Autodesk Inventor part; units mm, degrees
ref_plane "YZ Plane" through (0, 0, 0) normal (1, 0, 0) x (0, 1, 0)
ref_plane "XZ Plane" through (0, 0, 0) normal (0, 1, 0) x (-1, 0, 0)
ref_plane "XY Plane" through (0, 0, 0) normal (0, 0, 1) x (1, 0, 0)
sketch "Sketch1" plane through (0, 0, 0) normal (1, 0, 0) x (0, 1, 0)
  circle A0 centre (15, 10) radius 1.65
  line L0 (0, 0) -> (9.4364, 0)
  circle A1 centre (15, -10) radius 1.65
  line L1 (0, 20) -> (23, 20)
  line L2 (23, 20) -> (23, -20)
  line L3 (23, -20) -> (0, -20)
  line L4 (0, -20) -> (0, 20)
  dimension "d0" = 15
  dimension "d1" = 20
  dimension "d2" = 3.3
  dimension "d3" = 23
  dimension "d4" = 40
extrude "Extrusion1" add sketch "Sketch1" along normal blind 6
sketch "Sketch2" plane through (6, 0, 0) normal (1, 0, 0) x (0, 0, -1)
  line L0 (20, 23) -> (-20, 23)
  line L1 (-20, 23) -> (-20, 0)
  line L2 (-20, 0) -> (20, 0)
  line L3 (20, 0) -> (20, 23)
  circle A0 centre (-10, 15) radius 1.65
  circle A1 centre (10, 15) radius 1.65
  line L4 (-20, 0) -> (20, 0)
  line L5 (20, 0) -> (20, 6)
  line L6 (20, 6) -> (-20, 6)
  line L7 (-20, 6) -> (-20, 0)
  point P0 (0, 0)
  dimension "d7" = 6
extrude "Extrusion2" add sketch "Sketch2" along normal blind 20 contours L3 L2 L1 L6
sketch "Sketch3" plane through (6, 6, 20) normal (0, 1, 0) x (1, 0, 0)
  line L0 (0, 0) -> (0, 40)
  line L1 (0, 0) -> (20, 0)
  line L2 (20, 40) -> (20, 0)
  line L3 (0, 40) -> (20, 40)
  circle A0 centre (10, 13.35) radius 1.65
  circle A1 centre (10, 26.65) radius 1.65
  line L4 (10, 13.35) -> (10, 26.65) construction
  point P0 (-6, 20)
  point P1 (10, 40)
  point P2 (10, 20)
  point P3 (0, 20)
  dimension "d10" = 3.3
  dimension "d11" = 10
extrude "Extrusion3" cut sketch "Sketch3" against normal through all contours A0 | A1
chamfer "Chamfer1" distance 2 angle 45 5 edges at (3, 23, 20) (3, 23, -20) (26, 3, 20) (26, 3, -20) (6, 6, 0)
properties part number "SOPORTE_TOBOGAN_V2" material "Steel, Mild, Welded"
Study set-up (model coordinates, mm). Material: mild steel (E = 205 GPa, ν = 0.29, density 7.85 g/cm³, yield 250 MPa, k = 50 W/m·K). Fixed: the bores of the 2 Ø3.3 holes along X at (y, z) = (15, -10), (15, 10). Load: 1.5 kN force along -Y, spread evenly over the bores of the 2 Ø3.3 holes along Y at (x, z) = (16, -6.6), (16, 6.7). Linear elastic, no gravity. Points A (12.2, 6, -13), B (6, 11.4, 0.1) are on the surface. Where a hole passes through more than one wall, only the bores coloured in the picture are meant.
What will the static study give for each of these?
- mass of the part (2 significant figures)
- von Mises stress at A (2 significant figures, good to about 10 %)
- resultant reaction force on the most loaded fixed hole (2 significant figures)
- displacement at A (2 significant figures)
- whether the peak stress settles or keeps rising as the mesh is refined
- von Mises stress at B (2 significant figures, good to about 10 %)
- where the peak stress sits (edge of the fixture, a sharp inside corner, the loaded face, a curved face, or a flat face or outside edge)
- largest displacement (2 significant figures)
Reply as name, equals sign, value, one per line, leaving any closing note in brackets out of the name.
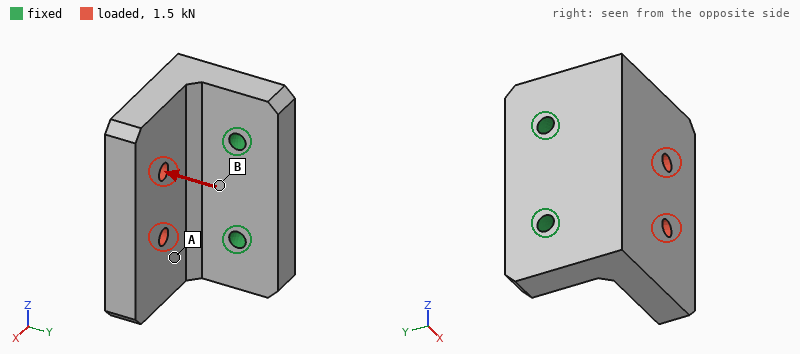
mass of the part = 80 g
von Mises stress at A = 25 MPa
resultant reaction force on the most loaded fixed hole = 770 N
displacement at A = 17 µm
whether the peak stress settles or keeps rising as the mesh is refined = keeps rising
von Mises stress at B = 63 MPa
where the peak stress sits = edge of the fixture
largest displacement = 48 µm
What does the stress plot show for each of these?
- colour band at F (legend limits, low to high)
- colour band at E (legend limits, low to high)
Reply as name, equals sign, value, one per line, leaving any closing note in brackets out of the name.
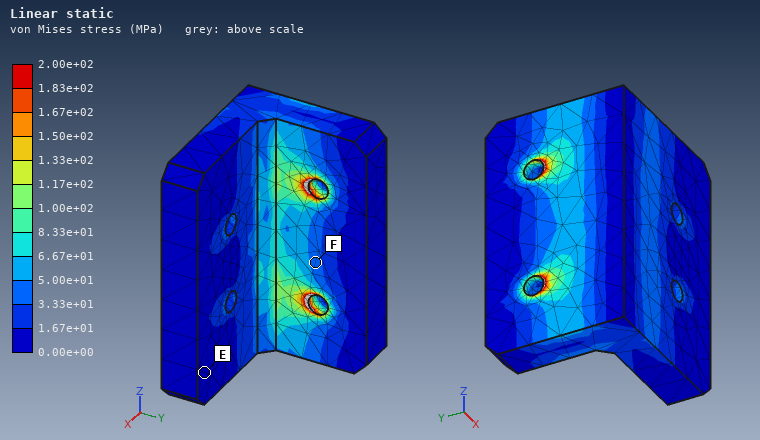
colour band at F = 3.33e+01 to 5.00e+01 MPa
colour band at E = 0.00e+00 to 1.67e+01 MPa
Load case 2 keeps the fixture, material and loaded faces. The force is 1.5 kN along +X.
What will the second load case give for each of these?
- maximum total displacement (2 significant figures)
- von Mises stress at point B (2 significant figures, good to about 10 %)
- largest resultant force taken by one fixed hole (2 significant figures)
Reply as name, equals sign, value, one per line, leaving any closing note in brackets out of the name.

maximum total displacement = 24 µm
von Mises stress at point B = 33 MPa
largest resultant force taken by one fixed hole = 750 N
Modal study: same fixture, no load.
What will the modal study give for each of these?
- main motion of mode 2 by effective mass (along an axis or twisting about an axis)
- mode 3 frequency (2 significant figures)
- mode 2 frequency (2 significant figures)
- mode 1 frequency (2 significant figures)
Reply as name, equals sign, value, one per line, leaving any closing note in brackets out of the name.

main motion of mode 2 by effective mass = along Z
mode 3 frequency = 14 kHz
mode 2 frequency = 8800 Hz
mode 1 frequency = 5200 Hz
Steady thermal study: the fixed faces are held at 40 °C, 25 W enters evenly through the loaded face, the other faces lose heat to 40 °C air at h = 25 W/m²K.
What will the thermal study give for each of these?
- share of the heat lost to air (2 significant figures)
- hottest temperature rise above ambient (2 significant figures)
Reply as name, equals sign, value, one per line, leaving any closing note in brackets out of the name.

share of the heat lost to air = 10 %
hottest temperature rise above ambient = 53 K
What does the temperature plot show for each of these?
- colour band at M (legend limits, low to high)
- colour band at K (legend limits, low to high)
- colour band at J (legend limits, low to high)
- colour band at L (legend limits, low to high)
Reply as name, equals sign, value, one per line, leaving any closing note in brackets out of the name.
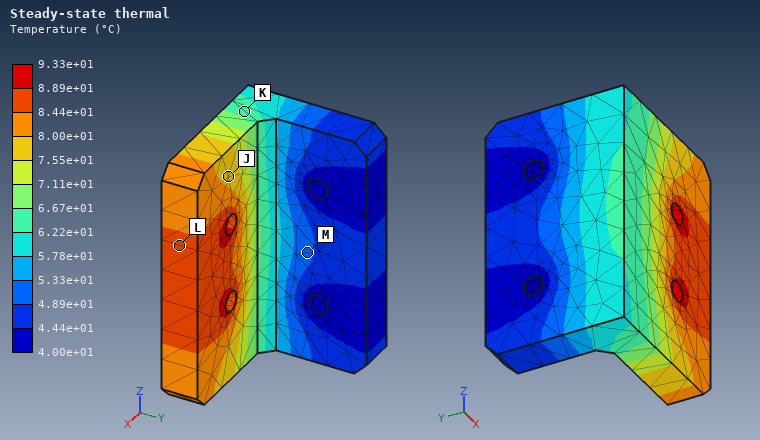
colour band at M = 4.89e+01 to 5.33e+01 °C
colour band at K = 6.22e+01 to 6.67e+01 °C
colour band at J = 7.55e+01 to 8.00e+01 °C
colour band at L = 8.44e+01 to 8.89e+01 °C
